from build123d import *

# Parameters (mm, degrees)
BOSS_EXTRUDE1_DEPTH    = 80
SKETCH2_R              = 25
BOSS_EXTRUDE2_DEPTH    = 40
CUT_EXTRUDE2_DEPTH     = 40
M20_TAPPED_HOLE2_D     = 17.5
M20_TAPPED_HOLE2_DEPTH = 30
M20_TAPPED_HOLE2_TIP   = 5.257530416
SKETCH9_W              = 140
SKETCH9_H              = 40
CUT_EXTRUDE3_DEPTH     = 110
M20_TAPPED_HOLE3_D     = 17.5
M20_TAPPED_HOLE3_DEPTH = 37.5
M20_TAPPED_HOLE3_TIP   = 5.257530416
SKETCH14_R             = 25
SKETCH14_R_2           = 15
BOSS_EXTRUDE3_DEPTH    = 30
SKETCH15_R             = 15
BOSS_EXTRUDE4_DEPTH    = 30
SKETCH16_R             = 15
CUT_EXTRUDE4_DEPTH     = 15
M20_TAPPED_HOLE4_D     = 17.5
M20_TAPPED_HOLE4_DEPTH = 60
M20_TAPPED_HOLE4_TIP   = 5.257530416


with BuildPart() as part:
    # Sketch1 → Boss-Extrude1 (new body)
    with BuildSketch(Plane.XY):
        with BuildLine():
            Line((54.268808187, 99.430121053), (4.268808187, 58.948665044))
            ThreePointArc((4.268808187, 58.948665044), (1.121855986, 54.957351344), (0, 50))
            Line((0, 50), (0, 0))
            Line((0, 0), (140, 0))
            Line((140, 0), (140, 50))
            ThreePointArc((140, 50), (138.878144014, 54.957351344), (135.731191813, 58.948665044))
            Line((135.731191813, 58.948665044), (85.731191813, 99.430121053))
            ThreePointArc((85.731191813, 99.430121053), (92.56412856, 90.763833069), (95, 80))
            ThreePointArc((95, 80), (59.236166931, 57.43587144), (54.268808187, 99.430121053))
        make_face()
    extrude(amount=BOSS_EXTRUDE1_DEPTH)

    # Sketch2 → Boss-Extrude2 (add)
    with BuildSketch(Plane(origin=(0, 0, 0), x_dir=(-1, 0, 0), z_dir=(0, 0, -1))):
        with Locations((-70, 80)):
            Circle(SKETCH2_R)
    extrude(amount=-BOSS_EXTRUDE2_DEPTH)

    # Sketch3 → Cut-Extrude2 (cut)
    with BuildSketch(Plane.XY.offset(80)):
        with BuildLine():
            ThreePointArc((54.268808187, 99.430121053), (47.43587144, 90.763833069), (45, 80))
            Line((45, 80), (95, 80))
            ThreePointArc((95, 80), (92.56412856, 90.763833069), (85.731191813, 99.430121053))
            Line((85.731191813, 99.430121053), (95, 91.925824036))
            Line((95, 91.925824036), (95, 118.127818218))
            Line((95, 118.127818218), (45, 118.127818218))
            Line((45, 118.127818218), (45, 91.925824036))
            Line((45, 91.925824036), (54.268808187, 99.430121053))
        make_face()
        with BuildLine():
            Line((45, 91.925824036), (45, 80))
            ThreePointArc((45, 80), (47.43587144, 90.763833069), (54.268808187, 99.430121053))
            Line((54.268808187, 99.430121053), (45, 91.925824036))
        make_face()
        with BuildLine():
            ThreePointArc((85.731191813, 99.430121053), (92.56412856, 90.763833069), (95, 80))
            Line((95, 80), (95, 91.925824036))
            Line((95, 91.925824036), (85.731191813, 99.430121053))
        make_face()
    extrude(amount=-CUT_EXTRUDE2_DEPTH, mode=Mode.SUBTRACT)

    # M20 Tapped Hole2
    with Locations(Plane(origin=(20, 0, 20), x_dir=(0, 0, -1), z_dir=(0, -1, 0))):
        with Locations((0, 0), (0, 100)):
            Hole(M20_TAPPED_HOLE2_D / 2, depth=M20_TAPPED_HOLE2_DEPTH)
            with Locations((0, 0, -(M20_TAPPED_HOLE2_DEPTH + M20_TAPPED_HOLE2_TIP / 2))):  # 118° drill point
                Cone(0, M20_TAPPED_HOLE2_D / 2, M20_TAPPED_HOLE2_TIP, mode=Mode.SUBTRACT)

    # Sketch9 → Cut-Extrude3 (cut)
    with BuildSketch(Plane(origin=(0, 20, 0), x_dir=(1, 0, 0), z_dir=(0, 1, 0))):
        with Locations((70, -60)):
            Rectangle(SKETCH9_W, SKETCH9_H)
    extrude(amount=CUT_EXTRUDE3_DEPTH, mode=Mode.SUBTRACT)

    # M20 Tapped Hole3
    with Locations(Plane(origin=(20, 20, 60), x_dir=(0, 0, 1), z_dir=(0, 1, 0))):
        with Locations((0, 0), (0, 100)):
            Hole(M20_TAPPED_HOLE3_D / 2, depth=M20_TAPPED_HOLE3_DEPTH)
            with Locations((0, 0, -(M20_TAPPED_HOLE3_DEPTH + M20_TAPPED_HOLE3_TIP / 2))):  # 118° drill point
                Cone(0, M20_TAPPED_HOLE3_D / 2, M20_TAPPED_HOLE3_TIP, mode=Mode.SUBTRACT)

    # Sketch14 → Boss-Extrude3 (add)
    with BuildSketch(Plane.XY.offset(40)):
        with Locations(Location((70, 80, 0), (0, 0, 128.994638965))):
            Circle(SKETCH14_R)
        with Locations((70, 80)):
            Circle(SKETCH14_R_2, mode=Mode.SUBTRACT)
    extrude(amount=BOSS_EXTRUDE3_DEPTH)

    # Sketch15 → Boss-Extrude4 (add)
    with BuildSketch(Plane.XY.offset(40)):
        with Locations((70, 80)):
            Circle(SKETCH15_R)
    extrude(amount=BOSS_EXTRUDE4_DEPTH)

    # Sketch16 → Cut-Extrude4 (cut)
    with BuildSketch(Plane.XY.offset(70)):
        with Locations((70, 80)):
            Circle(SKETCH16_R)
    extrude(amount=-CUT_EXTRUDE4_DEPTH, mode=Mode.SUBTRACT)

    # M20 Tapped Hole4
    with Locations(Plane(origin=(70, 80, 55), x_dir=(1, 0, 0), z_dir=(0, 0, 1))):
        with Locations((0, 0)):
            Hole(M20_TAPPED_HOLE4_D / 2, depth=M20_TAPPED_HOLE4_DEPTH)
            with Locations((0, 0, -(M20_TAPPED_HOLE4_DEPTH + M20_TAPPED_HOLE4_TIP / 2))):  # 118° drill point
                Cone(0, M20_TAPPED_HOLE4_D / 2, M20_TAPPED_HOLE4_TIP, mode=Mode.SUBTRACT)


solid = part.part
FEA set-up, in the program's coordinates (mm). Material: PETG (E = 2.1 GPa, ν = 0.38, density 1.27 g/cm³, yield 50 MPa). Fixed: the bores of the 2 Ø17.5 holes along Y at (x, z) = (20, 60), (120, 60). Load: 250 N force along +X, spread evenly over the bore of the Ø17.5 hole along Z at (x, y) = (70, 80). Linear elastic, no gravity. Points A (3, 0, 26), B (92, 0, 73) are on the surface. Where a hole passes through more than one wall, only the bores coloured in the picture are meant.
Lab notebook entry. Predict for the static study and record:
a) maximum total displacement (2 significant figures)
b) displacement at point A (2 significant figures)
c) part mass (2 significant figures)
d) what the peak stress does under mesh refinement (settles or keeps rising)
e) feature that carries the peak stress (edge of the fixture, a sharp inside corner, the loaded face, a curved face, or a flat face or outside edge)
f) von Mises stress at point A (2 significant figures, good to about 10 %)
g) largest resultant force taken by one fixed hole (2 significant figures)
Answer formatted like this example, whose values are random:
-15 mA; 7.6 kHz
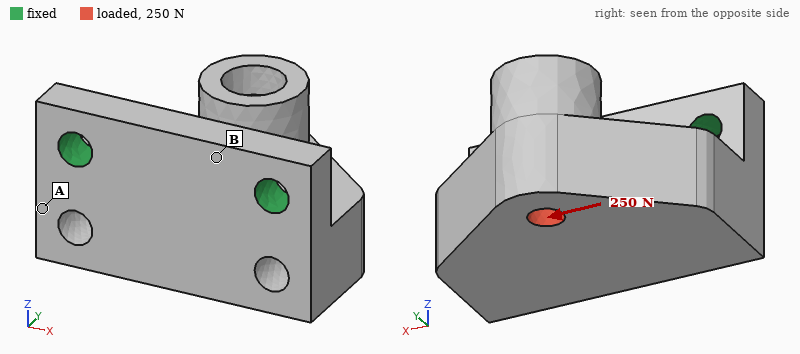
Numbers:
44 µm; 17 µm; 750 g; keeps rising; edge of the fixture; 0.26 MPa; 220 N
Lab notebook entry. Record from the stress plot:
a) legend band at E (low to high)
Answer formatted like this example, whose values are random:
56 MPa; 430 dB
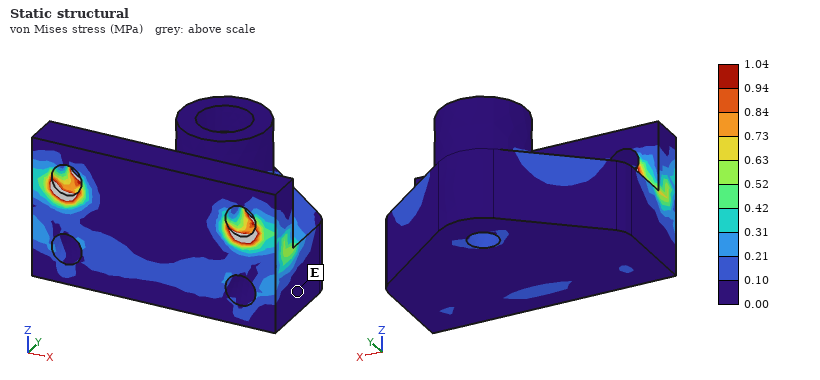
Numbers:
0.00 to 0.10 MPa
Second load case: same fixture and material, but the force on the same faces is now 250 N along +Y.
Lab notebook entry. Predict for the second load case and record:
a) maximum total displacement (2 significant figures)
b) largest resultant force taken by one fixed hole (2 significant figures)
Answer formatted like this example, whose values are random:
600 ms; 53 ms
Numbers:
75 µm; 130 N
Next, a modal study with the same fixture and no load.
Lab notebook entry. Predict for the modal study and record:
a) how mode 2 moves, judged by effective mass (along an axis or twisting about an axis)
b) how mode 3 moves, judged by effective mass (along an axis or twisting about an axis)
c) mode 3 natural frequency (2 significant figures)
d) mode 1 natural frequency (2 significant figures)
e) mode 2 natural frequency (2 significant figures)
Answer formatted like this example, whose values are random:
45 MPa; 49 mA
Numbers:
along X; along Y; 1100 Hz; 300 Hz; 770 Hz
